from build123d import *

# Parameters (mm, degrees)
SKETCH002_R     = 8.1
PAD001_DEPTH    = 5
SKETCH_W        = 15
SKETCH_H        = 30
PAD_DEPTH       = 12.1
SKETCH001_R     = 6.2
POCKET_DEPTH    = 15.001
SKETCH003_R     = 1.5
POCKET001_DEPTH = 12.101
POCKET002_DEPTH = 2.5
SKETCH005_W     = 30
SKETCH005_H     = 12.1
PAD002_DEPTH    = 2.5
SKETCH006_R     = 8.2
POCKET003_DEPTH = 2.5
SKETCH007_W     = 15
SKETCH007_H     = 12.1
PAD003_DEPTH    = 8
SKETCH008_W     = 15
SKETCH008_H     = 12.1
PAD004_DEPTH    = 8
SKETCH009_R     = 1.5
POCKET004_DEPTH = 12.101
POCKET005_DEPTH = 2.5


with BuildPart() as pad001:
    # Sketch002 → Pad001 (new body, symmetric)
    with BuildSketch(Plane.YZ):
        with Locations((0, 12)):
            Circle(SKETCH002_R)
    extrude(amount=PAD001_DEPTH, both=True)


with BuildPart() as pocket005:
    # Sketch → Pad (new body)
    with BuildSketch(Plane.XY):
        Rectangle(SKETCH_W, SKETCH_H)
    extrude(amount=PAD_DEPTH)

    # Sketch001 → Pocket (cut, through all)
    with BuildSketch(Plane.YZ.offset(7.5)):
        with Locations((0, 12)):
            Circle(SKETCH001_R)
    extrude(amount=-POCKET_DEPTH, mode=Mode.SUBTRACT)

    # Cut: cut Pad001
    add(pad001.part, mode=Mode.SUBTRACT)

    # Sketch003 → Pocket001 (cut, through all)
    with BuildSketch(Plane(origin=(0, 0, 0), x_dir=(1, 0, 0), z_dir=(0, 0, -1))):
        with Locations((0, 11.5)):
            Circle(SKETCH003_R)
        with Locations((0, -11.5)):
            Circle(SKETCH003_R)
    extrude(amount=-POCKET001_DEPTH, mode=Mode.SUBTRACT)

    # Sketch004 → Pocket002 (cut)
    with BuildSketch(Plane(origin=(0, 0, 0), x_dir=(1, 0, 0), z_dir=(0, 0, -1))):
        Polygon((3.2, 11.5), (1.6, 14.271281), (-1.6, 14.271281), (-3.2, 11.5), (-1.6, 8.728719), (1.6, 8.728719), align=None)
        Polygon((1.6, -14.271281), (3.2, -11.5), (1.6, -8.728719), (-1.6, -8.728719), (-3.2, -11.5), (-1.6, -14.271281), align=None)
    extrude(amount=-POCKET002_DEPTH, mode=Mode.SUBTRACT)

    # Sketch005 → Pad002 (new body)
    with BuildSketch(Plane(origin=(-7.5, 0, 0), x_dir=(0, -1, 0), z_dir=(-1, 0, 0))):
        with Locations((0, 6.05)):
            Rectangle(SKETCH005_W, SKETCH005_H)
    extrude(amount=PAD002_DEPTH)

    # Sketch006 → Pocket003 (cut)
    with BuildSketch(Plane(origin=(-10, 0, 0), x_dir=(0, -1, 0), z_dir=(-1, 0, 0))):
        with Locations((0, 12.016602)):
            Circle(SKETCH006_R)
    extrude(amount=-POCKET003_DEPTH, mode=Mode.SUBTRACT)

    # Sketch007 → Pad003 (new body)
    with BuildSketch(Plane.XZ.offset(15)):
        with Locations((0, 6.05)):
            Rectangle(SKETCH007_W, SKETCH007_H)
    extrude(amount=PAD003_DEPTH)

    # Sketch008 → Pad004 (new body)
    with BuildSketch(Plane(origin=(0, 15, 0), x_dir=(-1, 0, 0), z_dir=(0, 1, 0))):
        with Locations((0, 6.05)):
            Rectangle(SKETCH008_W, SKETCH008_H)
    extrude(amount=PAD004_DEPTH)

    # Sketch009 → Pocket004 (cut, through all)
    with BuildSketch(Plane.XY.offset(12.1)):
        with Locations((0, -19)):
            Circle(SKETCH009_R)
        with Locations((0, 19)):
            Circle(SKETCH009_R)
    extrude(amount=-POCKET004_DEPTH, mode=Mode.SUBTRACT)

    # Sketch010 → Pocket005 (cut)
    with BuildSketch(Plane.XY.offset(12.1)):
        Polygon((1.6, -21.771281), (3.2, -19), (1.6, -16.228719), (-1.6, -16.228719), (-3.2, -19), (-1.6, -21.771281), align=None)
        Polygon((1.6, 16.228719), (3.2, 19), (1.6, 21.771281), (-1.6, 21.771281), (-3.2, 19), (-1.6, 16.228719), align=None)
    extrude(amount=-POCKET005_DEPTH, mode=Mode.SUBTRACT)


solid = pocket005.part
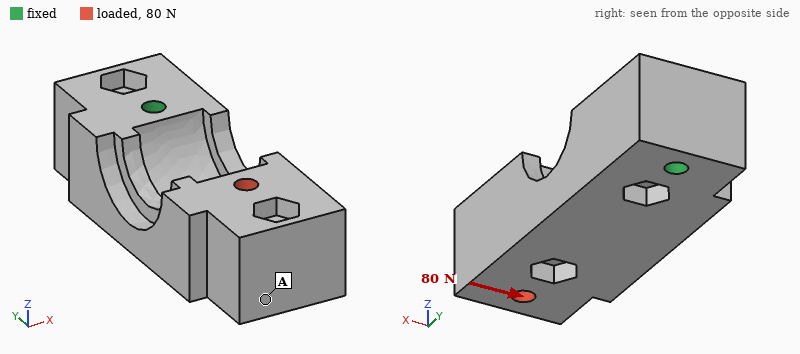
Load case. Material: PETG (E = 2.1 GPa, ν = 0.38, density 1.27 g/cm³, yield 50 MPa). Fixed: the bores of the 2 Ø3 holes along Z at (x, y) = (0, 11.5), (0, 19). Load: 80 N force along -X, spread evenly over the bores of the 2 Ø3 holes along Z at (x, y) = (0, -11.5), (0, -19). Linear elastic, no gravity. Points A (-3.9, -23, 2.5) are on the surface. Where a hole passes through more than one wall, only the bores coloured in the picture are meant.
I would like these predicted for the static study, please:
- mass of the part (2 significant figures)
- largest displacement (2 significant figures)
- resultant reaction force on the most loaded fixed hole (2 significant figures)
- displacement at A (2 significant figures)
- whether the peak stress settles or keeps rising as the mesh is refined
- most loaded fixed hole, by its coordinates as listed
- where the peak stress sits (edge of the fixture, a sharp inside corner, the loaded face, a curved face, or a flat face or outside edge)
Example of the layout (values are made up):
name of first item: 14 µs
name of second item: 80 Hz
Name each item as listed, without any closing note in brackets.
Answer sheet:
mass of the part: 9.0 g
largest displacement: 0.35 mm
resultant reaction force on the most loaded fixed hole: 270 N
displacement at A: 0.28 mm
whether the peak stress settles or keeps rising as the mesh is refined: keeps rising
most loaded fixed hole, by its coordinates as listed: (0, 11.5)
where the peak stress sits: edge of the fixture
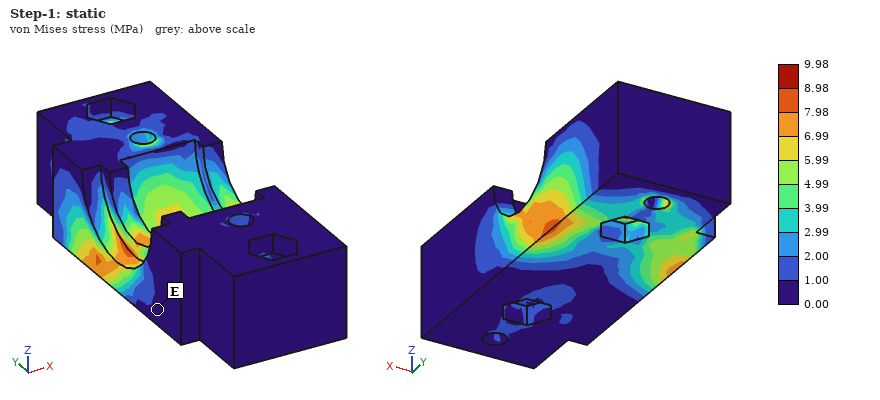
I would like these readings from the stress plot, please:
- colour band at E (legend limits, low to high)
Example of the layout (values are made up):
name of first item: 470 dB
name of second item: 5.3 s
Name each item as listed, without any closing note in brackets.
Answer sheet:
colour band at E: 0.00 to 1.00 MPa
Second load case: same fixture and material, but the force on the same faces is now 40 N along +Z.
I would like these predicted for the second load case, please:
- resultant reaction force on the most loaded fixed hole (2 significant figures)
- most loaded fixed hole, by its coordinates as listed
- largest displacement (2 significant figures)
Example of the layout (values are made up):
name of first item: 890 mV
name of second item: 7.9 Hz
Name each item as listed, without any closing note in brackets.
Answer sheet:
resultant reaction force on the most loaded fixed hole: 86 N
most loaded fixed hole, by its coordinates as listed: (0, 11.5)
largest displacement: 0.58 mm
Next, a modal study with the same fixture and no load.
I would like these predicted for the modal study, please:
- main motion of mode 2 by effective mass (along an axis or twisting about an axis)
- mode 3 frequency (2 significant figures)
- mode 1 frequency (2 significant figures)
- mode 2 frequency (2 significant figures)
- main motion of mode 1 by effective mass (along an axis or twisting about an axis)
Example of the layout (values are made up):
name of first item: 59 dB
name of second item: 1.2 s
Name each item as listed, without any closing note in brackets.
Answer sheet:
main motion of mode 2 by effective mass: along X
mode 3 frequency: 2800 Hz
mode 1 frequency: 820 Hz
mode 2 frequency: 1500 Hz
main motion of mode 1 by effective mass: along Z
